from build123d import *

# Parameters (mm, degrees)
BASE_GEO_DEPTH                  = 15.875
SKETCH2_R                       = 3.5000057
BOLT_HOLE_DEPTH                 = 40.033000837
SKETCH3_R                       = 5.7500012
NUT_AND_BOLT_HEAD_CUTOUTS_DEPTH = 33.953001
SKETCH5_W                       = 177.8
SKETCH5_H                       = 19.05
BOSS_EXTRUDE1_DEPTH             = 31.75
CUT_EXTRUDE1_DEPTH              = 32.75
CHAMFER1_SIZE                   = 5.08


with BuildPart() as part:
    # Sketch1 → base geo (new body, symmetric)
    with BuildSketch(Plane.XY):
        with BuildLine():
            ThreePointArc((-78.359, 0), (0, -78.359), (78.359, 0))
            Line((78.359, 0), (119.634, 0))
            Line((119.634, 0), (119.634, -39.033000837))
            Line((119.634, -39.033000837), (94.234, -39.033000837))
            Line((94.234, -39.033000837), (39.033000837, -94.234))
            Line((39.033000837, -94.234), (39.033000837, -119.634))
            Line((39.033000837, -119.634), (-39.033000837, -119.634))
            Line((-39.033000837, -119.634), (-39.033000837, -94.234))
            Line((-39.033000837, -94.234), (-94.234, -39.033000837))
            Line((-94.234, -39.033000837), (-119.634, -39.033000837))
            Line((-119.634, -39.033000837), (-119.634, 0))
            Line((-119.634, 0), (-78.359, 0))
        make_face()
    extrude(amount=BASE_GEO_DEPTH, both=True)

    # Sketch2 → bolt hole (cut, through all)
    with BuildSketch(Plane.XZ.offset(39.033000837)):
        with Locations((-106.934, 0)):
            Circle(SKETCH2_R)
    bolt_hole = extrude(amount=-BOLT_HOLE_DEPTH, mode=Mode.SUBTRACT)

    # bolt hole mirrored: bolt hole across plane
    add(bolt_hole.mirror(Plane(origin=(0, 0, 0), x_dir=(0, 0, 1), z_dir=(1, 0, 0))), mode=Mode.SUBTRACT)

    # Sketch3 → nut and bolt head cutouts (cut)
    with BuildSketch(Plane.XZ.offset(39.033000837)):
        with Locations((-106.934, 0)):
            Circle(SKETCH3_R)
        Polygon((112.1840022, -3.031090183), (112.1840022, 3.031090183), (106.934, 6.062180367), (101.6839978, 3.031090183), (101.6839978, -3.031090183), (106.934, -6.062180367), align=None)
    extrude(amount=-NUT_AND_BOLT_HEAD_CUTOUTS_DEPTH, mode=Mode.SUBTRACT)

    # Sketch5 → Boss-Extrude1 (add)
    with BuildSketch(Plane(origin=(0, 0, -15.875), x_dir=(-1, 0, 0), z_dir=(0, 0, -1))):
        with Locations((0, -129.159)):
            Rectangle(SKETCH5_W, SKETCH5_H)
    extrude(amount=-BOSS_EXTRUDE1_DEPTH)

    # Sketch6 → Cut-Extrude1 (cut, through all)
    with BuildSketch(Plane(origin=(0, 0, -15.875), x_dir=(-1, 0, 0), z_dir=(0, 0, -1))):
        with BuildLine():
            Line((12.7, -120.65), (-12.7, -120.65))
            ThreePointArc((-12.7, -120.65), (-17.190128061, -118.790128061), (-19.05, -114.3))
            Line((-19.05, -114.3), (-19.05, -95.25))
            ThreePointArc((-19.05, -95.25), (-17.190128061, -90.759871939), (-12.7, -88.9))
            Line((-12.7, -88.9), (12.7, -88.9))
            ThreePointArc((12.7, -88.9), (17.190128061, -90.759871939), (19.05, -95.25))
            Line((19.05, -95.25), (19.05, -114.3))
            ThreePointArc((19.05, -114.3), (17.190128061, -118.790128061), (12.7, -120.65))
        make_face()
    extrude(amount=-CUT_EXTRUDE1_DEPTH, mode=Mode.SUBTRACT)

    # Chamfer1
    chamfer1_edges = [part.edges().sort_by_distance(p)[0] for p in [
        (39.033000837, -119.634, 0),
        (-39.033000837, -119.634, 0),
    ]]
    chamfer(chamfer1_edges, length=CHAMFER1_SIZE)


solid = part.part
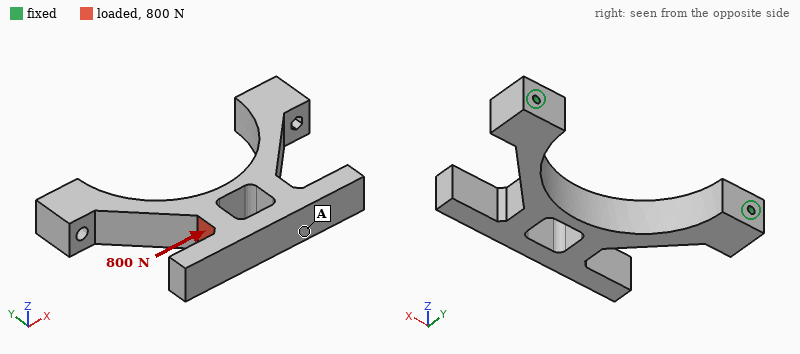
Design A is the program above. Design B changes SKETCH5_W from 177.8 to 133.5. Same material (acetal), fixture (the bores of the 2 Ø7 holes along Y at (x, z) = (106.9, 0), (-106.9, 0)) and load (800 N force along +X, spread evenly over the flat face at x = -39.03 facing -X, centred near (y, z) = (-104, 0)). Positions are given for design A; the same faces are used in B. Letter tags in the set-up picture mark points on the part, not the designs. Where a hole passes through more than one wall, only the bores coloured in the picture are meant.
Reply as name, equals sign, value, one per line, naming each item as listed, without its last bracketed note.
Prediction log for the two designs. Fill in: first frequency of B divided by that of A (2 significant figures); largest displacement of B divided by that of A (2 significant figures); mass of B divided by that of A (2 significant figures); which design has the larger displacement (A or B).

first frequency of B divided by that of A = 1.1
largest displacement of B divided by that of A = 0.81
mass of B divided by that of A = 0.92
which design has the larger displacement = A
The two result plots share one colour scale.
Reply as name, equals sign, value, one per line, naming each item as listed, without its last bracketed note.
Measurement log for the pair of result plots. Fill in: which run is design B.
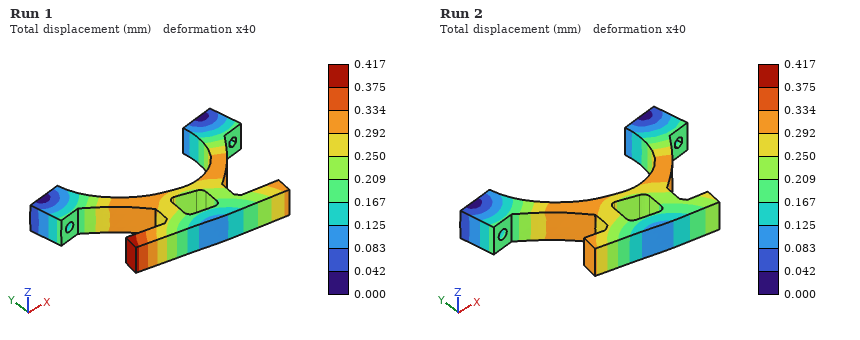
which run is design B = Run 2
